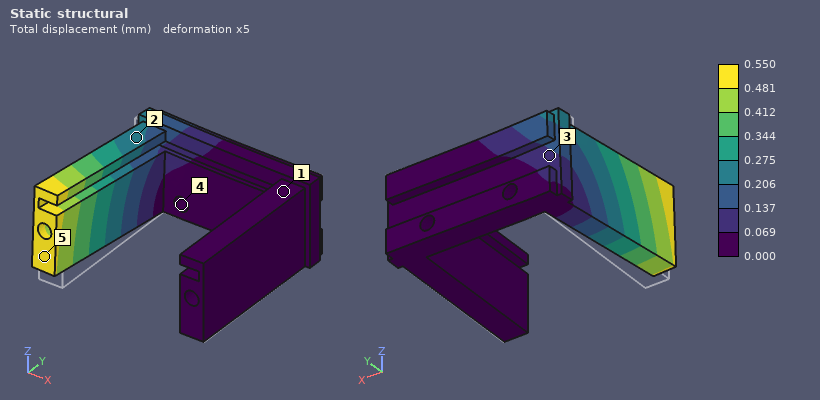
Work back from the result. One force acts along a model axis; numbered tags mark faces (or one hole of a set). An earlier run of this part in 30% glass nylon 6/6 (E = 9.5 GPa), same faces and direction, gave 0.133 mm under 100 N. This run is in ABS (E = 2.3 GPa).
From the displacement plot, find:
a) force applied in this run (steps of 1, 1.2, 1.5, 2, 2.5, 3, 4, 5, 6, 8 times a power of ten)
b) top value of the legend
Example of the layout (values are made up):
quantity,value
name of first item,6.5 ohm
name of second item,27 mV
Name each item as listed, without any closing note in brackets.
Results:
quantity,value
force applied in this run,100 N
top value of the legend,0.550 mm
